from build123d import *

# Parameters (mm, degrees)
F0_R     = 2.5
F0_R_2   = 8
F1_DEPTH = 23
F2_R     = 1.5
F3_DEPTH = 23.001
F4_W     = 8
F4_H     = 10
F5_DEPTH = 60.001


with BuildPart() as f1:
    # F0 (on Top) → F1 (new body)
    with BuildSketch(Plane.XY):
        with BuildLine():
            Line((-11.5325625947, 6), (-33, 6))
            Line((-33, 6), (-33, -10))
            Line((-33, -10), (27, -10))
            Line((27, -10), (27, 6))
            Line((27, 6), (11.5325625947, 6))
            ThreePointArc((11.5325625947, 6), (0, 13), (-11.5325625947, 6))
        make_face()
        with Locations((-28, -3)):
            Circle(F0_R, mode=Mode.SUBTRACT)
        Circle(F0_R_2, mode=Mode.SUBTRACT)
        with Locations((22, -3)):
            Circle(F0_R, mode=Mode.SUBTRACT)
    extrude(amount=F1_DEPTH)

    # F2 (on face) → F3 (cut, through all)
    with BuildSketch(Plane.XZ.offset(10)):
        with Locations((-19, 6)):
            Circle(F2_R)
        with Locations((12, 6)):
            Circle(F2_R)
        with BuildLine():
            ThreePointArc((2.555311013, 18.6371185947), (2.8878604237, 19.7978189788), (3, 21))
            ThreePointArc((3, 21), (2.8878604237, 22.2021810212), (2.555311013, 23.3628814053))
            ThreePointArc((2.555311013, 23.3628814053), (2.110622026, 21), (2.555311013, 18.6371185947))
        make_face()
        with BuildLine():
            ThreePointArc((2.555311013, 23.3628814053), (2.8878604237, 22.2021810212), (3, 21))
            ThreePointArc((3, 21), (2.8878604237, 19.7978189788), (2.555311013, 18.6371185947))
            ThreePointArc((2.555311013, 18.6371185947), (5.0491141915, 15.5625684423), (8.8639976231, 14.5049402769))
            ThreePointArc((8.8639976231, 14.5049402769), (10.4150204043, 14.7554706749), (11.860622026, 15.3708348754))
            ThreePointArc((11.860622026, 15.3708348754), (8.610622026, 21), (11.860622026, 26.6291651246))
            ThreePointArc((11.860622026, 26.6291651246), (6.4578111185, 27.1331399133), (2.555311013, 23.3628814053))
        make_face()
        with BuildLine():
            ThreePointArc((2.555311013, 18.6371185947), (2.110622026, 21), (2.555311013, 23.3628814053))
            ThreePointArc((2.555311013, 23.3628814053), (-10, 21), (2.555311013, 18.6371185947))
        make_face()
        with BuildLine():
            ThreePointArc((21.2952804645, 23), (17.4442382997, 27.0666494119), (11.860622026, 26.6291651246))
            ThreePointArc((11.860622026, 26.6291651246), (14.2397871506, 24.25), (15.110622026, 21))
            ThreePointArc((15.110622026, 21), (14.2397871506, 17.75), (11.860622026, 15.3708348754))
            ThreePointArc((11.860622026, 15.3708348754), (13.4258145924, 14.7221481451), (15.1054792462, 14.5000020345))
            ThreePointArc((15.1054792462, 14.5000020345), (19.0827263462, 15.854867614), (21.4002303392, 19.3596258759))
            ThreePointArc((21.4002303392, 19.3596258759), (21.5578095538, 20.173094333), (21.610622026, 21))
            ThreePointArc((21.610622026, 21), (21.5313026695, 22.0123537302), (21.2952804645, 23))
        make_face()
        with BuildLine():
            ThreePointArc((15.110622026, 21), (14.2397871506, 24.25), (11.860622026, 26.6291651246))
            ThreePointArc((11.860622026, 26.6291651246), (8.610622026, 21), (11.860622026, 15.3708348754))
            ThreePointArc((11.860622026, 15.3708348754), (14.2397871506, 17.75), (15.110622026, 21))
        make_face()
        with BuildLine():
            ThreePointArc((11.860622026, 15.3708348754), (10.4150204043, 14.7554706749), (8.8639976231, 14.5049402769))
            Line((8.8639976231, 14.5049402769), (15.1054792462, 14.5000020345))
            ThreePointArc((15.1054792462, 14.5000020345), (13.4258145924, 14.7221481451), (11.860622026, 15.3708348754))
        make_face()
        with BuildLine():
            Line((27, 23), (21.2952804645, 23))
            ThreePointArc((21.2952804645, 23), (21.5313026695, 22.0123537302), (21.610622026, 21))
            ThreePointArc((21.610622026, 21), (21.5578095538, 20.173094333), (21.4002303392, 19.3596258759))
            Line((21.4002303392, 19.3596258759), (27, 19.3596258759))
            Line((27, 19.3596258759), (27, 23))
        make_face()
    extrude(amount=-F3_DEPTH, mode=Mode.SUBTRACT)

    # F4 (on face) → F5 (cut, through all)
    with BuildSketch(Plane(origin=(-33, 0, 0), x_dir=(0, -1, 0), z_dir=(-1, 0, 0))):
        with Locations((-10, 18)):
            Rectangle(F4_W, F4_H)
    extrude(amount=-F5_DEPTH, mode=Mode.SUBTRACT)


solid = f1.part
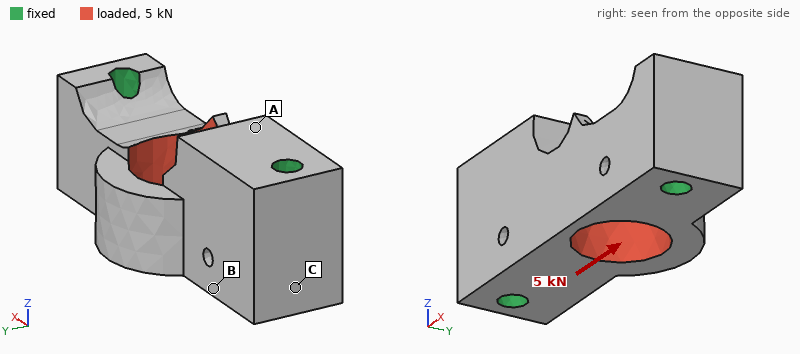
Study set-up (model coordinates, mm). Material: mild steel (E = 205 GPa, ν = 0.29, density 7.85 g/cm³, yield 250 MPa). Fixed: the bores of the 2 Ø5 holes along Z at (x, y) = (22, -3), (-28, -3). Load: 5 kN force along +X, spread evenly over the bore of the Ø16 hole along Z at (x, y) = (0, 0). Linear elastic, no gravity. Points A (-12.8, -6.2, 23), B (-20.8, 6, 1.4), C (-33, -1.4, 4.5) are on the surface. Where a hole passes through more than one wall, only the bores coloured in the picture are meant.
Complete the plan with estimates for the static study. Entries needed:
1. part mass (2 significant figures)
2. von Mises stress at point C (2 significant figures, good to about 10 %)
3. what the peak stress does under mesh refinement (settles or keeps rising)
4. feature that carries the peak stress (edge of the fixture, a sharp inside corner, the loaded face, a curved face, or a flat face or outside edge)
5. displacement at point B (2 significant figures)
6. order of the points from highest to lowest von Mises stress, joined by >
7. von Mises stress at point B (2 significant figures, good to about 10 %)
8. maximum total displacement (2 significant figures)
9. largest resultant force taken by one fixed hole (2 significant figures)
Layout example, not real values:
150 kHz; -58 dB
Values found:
120 g; 6.8 MPa; keeps rising; a sharp inside corner; 0.81 µm; B > C > A; 10 MPa; 2.3 µm; 2.5 kN
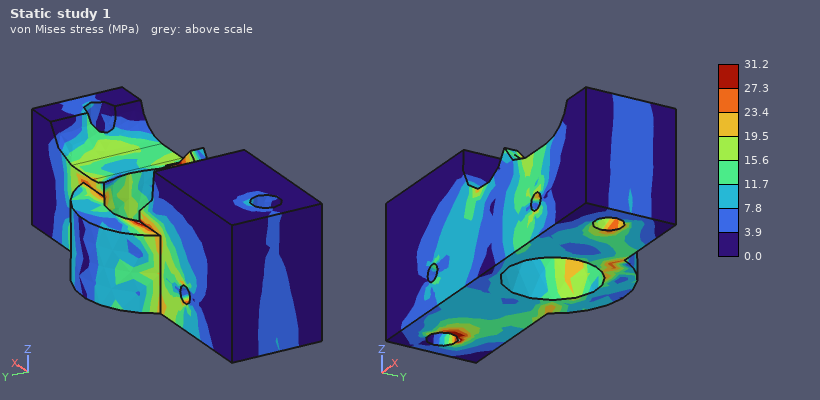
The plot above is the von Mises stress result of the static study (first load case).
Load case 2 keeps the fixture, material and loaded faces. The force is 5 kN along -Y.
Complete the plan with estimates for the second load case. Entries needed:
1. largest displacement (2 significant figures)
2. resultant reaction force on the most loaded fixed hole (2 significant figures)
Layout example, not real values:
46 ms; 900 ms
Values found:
9.2 µm; 2.6 kN
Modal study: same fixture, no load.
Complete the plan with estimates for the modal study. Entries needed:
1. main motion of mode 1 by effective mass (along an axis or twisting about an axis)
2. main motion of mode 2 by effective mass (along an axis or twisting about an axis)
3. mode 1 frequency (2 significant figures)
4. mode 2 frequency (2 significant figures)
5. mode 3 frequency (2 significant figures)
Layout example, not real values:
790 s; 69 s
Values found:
along Y; along Z; 19 kHz; 23 kHz; 29 kHz
